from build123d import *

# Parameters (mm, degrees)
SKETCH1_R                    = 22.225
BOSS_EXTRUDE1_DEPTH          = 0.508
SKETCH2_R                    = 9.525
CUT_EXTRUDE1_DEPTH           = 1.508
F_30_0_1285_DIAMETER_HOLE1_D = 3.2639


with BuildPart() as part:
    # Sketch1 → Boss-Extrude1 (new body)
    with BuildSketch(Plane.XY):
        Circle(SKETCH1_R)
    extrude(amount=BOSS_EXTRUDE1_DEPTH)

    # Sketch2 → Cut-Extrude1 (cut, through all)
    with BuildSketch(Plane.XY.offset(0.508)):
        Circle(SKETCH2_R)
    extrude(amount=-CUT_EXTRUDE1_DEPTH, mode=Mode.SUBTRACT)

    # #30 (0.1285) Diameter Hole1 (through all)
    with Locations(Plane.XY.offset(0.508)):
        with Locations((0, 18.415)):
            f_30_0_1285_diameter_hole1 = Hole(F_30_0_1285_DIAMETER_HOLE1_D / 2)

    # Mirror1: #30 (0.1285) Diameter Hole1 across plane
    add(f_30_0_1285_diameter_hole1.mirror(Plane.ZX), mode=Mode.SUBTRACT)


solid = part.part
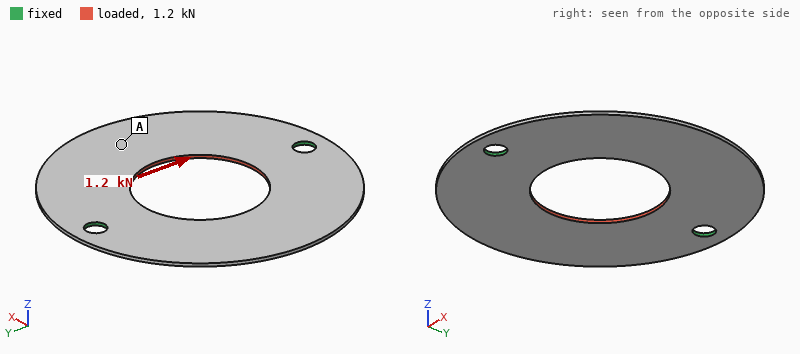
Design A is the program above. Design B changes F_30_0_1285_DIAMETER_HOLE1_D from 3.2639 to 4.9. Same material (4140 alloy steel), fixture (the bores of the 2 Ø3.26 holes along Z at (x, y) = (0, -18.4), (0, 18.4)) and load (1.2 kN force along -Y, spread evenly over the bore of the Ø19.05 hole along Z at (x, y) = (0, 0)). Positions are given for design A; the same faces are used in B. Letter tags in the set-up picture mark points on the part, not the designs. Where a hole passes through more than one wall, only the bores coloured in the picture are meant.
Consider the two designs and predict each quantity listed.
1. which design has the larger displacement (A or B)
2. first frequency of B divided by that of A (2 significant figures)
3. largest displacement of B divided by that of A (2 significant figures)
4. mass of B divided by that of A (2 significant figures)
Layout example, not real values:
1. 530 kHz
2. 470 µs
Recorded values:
1. A
2. 1.1
3. 0.89
4. 0.98
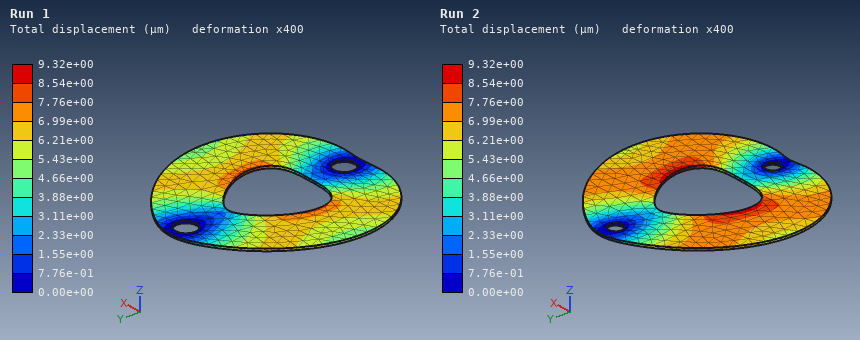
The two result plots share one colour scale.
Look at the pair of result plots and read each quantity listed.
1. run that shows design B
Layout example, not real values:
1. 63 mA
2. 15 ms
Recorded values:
1. Run 1
